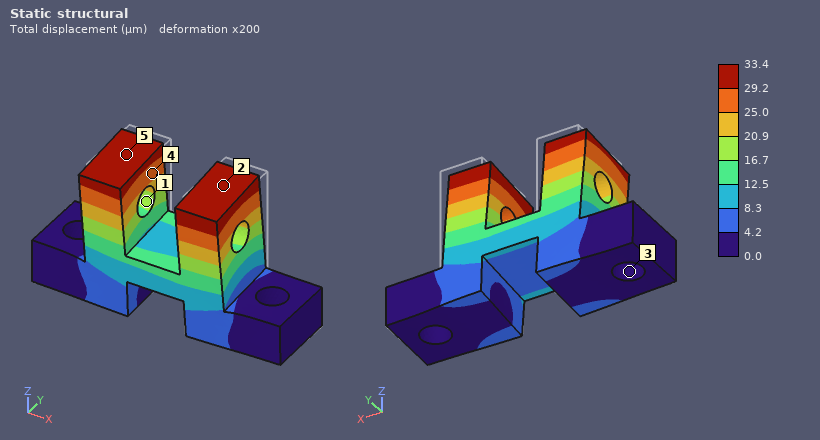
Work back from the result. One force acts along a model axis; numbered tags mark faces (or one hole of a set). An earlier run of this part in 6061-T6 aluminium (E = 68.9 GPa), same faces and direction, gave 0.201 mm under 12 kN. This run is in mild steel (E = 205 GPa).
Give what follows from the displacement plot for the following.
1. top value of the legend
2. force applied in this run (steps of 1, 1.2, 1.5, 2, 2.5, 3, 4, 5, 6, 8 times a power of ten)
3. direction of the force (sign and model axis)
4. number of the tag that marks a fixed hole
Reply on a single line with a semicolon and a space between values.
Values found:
33.4 µm; 6 kN; -Y; 3
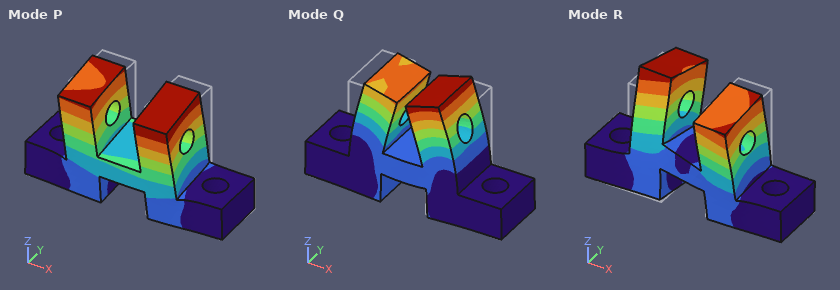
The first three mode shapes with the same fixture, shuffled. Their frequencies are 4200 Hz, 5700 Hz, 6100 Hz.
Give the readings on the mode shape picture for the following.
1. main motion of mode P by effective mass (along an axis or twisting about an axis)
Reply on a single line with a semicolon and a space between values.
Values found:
along Y
